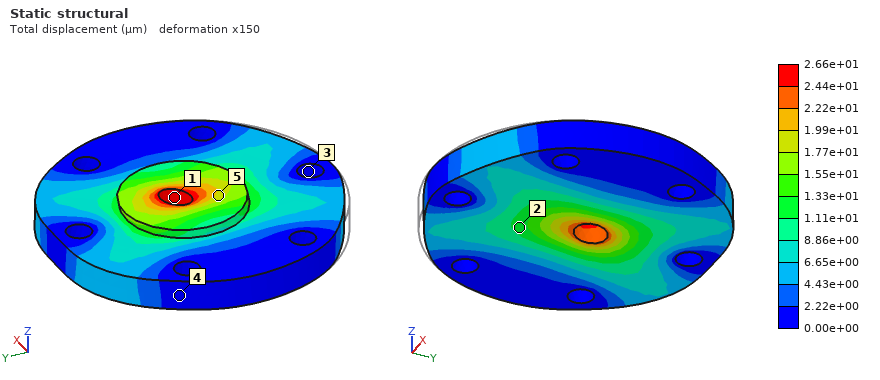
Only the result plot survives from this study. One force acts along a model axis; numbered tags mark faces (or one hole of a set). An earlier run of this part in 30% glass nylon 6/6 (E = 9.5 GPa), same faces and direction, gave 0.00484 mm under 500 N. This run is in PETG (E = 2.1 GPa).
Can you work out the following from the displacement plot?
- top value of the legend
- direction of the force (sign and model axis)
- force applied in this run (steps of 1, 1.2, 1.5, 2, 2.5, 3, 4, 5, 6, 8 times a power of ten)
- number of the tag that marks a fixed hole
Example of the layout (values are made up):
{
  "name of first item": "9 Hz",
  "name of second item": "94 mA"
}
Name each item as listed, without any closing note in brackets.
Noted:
{
  "top value of the legend": "2.66e+01 µm",
  "direction of the force": "+Y",
  "force applied in this run": "600 N",
  "number of the tag that marks a fixed hole": "3"
}
